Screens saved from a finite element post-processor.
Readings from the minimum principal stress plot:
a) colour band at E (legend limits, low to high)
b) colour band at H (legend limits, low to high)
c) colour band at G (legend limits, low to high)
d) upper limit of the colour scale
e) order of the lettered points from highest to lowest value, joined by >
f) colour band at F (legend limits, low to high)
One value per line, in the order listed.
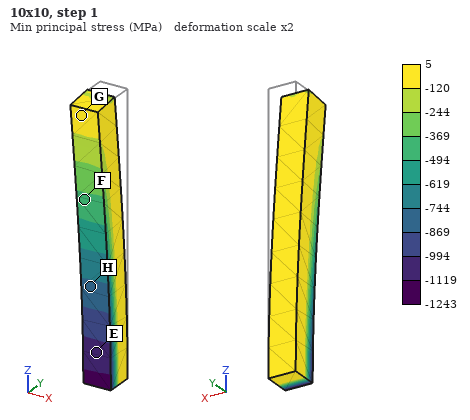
-1119 to -994 MPa
-869 to -744 MPa
-120 to 5 MPa
5 MPa
G > F > H > E
-494 to -369 MPa
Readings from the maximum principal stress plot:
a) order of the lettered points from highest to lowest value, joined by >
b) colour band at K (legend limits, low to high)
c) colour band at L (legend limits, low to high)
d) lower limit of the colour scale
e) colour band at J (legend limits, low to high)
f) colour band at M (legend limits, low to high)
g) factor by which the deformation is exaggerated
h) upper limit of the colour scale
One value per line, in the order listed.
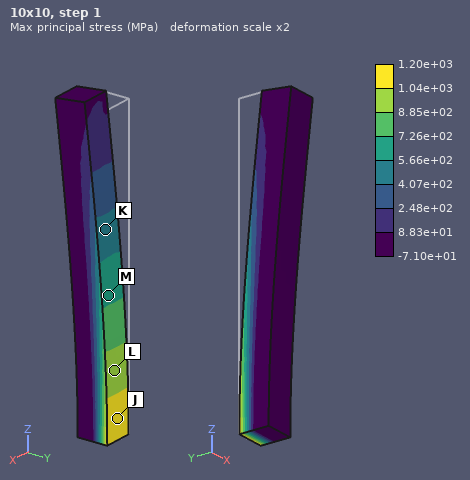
J > L > M > K
4.07e+02 to 5.66e+02 MPa
8.85e+02 to 1.04e+03 MPa
-7.10e+01 MPa
1.04e+03 to 1.20e+03 MPa
5.66e+02 to 7.26e+02 MPa
2
1.20e+03 MPa
